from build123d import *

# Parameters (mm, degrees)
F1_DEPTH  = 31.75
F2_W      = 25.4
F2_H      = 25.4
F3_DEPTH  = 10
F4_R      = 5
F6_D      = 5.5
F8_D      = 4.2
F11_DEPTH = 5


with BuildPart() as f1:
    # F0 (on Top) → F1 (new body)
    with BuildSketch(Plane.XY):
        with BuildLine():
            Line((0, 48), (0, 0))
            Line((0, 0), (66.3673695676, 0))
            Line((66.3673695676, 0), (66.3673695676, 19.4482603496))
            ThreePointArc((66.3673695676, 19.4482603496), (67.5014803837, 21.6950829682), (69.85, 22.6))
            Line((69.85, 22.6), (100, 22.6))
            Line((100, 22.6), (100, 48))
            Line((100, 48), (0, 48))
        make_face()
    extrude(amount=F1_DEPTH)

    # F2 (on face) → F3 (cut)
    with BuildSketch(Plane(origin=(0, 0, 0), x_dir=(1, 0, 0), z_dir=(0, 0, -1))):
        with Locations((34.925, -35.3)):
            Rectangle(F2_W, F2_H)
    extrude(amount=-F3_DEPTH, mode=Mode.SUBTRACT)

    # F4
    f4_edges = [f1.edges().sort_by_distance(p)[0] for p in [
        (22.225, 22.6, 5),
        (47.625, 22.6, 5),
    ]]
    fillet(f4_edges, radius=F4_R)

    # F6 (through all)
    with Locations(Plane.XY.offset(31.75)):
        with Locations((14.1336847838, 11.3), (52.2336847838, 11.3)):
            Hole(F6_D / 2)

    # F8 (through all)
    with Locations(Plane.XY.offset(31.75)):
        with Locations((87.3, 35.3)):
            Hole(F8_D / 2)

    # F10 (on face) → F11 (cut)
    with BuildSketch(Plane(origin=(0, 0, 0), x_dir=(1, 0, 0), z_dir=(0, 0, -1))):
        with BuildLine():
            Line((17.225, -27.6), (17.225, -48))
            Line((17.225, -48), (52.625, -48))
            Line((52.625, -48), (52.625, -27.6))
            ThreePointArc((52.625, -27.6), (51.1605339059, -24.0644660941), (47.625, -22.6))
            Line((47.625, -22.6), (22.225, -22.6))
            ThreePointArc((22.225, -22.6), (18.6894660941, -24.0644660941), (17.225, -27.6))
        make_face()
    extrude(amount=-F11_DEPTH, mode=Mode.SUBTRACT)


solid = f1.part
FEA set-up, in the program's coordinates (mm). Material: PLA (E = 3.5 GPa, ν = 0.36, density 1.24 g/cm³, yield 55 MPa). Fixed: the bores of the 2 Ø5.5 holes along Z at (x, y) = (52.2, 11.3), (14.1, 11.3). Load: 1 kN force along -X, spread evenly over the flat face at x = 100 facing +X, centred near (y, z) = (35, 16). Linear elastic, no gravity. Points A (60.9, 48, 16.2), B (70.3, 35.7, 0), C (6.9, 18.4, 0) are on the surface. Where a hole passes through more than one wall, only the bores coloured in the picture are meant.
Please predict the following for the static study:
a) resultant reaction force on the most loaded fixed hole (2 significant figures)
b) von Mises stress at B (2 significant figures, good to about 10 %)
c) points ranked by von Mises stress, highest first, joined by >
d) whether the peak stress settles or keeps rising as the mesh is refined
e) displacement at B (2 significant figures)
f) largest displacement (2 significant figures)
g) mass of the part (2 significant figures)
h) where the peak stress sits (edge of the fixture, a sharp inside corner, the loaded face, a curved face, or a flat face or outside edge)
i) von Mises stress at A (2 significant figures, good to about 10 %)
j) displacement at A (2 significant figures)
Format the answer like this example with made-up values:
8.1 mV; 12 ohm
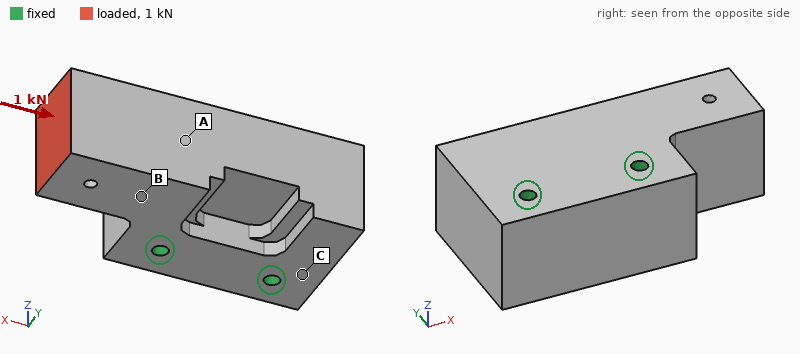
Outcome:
780 N; 0.94 MPa; A > B > C; keeps rising; 40 µm; 78 µm; 150 g; edge of the fixture; 2.0 MPa; 39 µm
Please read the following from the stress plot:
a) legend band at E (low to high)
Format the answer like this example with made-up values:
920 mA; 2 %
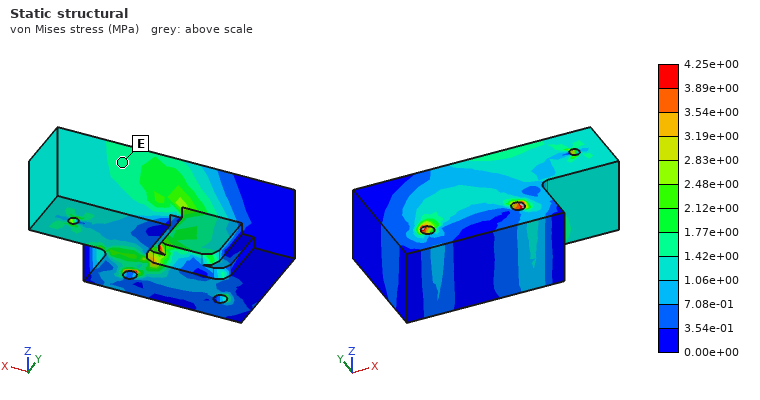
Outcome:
1.42e+00 to 1.77e+00 MPa
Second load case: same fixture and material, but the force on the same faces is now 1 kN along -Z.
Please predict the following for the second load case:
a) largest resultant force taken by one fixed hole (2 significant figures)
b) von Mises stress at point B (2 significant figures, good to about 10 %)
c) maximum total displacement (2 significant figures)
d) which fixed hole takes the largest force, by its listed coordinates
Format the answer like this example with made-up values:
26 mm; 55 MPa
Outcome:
1.5 kN; 5.5 MPa; 0.43 mm; (52.2, 11.3)
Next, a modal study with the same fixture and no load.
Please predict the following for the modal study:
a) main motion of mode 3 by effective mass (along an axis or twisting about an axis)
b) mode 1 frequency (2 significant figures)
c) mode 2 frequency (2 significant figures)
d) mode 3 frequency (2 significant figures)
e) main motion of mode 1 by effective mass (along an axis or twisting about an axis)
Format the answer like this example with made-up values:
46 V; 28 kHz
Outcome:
along Z; 1900 Hz; 2300 Hz; 3500 Hz; along Z
